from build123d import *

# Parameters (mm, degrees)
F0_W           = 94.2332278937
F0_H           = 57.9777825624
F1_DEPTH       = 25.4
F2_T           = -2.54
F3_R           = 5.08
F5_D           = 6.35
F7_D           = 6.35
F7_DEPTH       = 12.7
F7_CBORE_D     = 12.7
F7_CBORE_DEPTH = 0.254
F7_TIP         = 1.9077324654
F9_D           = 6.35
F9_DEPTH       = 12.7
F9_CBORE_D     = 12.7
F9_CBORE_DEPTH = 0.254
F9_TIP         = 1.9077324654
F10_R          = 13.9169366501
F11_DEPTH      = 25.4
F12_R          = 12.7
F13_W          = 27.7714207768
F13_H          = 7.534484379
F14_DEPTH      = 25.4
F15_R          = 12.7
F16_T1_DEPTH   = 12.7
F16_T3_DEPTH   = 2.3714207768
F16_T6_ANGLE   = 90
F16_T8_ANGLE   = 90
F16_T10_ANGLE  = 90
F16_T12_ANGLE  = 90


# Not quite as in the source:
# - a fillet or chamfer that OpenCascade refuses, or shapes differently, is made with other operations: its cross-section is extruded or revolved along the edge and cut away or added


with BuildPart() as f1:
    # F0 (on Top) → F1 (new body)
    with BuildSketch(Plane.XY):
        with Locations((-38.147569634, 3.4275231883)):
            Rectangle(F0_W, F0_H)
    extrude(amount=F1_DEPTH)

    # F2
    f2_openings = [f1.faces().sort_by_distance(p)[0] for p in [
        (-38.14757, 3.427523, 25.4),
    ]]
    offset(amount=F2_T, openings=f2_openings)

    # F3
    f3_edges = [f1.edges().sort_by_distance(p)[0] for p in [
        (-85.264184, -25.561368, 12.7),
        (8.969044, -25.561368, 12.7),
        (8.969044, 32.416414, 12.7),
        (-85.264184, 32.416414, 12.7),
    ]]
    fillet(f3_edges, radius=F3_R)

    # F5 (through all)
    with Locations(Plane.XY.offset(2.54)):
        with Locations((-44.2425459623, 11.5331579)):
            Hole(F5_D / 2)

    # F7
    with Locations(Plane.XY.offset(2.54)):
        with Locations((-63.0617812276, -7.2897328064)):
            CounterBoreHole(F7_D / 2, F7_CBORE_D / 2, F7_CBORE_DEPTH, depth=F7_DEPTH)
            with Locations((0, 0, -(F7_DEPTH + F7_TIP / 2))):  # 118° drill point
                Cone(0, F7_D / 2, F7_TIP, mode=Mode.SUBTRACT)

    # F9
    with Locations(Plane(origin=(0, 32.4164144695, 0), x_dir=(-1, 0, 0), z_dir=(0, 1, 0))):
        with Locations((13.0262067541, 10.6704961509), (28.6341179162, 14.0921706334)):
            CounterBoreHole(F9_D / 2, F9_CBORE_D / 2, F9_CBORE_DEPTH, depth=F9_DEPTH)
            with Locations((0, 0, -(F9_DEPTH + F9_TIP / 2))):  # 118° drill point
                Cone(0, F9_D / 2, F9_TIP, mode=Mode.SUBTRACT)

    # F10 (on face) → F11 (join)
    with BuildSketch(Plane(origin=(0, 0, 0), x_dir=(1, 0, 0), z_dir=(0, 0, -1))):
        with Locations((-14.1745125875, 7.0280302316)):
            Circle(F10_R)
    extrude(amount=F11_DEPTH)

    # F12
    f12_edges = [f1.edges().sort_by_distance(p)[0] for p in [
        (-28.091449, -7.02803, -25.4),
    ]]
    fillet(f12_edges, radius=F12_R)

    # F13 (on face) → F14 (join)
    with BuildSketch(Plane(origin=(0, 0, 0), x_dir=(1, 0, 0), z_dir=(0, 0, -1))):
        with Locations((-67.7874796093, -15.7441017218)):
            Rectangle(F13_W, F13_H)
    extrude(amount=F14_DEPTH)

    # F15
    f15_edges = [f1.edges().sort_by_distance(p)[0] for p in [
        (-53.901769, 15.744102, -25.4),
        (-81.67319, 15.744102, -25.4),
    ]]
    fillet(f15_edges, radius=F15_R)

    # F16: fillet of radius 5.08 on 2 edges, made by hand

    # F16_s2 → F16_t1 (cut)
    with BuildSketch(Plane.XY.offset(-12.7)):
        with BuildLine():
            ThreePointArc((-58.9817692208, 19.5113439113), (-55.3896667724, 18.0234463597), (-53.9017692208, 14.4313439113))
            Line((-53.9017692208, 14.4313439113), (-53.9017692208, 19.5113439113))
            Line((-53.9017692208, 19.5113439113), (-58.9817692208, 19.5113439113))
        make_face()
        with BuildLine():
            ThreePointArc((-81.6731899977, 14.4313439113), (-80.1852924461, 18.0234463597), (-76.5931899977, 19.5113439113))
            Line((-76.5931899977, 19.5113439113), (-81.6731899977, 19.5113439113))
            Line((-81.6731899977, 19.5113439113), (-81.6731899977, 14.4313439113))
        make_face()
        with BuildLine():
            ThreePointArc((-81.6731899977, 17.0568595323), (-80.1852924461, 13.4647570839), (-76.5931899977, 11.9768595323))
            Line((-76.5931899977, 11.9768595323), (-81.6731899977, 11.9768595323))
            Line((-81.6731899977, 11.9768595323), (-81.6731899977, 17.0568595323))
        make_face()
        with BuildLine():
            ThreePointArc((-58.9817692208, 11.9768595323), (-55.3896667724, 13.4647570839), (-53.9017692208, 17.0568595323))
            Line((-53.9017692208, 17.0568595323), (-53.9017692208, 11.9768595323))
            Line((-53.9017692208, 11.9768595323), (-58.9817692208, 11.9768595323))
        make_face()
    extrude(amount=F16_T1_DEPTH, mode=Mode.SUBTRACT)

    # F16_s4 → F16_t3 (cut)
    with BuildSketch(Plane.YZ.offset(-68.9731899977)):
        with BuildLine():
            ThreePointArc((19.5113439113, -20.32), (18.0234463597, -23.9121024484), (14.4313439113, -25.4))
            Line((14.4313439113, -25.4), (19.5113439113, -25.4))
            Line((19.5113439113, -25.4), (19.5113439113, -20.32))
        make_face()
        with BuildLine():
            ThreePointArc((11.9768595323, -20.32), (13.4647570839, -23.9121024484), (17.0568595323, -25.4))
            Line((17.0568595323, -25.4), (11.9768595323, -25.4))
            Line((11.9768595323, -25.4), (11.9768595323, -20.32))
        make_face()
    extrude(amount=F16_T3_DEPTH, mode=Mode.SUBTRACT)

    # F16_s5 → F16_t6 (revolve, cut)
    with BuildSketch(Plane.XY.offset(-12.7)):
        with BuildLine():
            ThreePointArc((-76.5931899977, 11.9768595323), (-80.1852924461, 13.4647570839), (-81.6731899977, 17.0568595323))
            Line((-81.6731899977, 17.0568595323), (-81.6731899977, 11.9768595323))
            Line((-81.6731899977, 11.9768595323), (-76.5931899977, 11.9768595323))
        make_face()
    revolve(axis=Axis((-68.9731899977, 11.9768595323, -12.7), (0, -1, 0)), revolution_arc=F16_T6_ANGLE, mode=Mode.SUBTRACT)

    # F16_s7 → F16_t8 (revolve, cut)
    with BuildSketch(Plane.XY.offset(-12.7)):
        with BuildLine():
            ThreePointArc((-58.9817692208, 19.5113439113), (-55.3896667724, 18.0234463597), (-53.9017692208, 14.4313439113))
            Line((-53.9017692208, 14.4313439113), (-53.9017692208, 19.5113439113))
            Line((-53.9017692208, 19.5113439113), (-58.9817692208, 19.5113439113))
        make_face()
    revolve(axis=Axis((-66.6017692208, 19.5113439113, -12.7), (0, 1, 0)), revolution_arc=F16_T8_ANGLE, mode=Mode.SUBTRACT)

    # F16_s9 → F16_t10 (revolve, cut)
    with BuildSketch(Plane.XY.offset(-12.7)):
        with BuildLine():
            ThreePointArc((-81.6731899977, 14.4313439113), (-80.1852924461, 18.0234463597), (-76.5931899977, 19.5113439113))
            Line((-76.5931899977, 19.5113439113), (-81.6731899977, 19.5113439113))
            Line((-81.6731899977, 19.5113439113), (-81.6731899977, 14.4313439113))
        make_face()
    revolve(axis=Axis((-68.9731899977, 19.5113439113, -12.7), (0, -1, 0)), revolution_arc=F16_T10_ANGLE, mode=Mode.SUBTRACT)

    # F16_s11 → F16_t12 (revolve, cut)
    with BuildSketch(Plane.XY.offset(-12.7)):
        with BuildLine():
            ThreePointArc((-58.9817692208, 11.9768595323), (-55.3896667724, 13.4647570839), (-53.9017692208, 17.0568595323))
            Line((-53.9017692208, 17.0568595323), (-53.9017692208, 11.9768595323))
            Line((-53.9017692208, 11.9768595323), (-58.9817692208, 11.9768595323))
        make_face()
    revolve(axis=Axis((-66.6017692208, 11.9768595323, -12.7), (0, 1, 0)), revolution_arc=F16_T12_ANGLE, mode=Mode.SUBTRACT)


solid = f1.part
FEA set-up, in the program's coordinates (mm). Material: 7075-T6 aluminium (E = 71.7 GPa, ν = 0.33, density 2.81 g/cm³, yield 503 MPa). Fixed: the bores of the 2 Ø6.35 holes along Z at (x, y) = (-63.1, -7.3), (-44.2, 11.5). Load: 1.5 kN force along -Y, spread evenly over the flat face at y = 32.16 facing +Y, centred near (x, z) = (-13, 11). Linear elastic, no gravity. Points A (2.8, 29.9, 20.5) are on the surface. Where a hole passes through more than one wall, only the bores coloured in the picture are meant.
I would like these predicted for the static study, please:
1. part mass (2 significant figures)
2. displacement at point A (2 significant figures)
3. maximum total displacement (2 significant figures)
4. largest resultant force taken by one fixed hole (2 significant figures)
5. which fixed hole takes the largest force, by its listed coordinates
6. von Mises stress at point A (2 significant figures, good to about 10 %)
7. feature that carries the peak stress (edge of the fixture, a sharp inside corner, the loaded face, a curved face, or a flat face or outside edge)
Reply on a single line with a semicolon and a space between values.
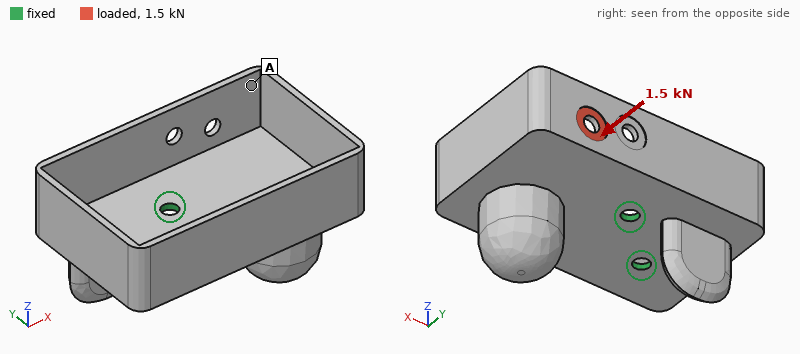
130 g; 0.49 mm; 0.76 mm; 2.6 kN; (-44.2, 11.5); 59 MPa; a curved face
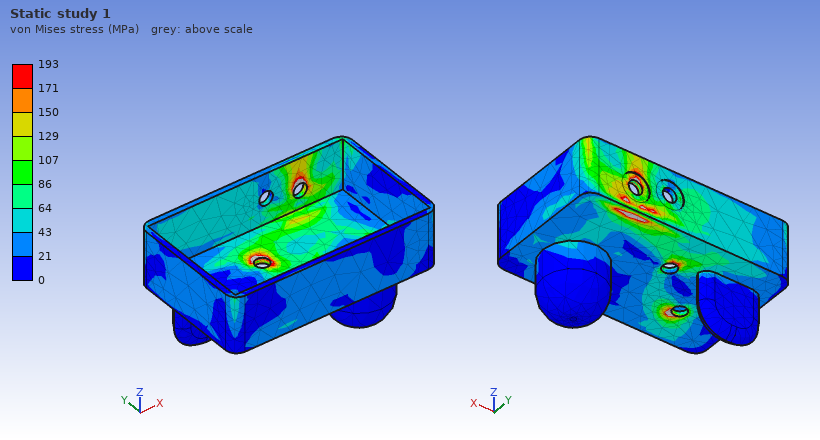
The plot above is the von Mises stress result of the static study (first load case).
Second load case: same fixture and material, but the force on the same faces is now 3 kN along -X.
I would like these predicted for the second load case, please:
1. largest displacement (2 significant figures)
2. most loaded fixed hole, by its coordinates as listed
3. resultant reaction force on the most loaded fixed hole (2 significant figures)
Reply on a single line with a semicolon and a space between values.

0.93 mm; (-44.2, 11.5); 4.4 kN
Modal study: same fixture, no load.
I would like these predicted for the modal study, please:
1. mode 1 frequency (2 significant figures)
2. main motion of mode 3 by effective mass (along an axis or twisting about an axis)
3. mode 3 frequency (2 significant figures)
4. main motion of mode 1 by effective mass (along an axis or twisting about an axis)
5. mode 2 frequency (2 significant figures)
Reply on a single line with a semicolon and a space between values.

480 Hz; along Z; 1300 Hz; along Z; 1100 Hz
